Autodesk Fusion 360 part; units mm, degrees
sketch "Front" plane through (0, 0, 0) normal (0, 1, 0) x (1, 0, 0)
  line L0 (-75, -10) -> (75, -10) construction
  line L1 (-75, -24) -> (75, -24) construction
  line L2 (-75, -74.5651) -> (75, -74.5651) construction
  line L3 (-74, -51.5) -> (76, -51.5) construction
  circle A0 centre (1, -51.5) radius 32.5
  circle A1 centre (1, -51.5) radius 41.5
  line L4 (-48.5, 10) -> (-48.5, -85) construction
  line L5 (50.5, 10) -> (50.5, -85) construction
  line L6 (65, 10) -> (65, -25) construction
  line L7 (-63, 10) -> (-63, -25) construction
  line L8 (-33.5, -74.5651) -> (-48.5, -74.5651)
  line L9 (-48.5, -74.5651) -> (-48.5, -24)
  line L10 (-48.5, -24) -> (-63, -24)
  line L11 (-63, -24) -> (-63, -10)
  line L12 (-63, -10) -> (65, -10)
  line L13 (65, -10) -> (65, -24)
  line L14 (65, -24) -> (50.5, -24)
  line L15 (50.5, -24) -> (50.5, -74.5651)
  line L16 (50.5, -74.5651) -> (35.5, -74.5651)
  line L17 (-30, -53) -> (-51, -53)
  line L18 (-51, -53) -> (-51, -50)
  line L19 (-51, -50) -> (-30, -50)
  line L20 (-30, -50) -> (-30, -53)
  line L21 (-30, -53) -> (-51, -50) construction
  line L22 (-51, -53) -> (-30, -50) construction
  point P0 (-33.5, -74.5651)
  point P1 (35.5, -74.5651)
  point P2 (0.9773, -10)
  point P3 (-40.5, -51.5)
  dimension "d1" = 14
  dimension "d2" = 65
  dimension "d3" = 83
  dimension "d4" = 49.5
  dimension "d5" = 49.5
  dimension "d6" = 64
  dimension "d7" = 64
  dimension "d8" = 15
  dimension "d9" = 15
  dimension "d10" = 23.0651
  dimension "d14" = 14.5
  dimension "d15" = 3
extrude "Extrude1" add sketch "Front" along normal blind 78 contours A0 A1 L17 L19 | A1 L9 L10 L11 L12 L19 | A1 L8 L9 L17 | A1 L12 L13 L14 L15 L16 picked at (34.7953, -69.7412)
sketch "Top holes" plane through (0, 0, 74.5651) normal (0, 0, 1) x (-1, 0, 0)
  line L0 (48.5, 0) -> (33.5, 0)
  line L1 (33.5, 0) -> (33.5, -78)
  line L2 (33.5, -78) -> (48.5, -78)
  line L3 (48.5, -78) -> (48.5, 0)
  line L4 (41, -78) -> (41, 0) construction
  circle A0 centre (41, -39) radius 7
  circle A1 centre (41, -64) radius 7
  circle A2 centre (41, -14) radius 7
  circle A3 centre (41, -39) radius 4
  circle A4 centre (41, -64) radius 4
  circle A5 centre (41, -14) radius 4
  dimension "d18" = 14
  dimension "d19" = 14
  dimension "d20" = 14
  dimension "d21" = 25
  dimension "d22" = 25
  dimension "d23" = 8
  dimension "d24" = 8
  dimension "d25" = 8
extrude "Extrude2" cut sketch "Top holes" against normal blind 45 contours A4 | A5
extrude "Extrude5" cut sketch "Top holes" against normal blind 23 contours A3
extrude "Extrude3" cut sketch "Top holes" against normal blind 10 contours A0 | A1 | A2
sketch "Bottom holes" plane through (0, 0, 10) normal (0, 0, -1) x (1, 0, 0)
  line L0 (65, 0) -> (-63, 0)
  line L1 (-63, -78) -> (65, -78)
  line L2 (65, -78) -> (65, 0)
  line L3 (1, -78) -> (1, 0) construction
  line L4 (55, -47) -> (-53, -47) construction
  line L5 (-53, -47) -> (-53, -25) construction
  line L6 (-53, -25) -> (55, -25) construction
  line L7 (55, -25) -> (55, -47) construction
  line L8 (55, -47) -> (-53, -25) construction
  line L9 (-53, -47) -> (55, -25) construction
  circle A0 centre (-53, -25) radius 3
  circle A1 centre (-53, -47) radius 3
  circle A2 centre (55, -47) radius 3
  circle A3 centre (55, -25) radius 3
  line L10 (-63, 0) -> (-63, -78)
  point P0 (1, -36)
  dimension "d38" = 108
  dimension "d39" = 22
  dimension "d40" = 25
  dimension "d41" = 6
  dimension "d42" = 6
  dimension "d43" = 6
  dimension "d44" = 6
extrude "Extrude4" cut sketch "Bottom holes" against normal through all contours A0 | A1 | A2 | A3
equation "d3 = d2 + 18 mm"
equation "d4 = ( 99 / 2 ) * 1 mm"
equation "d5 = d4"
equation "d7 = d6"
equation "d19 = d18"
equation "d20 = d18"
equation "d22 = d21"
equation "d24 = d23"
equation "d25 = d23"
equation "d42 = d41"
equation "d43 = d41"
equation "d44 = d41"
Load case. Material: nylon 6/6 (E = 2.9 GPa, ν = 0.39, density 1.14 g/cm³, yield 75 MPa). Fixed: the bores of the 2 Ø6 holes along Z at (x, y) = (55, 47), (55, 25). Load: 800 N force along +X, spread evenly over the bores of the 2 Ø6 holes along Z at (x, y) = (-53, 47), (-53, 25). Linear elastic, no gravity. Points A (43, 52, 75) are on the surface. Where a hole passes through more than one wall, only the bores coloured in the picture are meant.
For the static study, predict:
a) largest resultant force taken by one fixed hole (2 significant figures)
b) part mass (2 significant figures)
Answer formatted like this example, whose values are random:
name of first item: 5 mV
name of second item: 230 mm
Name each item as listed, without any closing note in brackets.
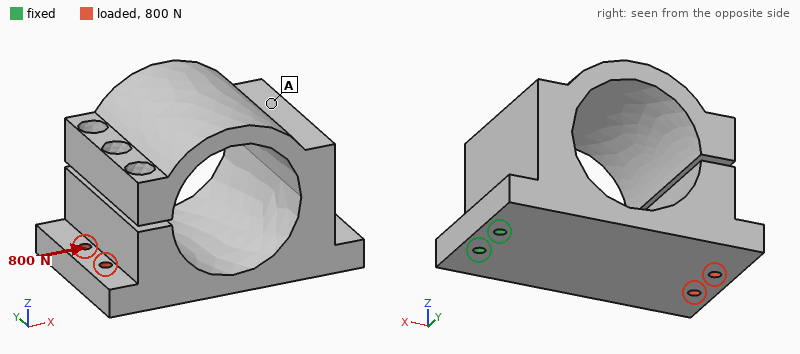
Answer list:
largest resultant force taken by one fixed hole: 400 N
part mass: 370 g
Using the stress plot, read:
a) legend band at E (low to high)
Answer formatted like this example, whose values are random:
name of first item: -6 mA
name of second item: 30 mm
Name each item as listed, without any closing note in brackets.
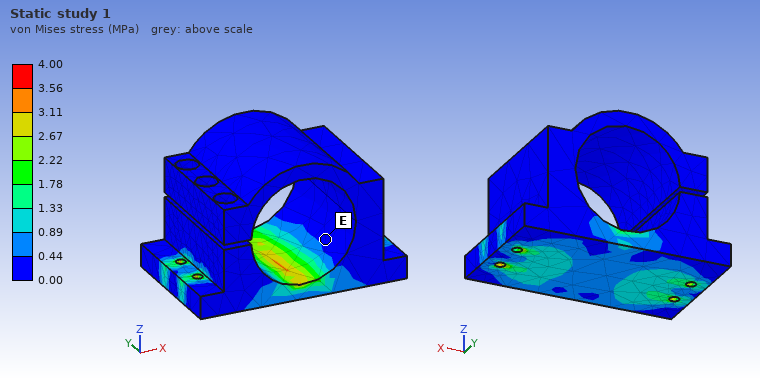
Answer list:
legend band at E: 0.00 to 0.44 MPa
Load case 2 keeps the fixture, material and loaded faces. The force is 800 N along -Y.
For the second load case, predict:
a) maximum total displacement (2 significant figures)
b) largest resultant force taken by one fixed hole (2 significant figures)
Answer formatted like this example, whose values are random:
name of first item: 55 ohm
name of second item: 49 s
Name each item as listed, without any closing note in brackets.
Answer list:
maximum total displacement: 0.96 mm
largest resultant force taken by one fixed hole: 3.2 kN
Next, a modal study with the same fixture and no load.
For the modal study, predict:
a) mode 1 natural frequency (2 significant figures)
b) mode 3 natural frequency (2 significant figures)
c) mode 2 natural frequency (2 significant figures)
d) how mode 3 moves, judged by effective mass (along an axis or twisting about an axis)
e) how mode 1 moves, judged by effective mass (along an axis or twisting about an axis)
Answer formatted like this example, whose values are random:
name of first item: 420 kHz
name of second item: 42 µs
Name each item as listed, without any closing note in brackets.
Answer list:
mode 1 natural frequency: 160 Hz
mode 3 natural frequency: 310 Hz
mode 2 natural frequency: 220 Hz
how mode 3 moves, judged by effective mass: along Y
how mode 1 moves, judged by effective mass: along Z
